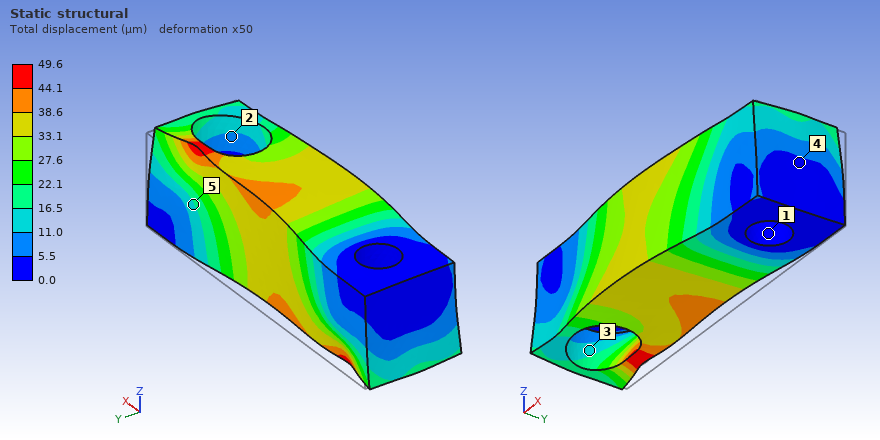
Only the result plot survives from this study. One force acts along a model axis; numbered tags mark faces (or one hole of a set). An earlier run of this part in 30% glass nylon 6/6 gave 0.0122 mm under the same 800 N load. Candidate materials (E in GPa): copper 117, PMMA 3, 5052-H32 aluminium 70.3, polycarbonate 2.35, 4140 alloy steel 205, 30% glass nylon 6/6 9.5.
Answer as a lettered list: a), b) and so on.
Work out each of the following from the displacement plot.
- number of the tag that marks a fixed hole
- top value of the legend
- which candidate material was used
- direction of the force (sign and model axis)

a) 1
b) 49.6 µm
c) polycarbonate
d) -Y
